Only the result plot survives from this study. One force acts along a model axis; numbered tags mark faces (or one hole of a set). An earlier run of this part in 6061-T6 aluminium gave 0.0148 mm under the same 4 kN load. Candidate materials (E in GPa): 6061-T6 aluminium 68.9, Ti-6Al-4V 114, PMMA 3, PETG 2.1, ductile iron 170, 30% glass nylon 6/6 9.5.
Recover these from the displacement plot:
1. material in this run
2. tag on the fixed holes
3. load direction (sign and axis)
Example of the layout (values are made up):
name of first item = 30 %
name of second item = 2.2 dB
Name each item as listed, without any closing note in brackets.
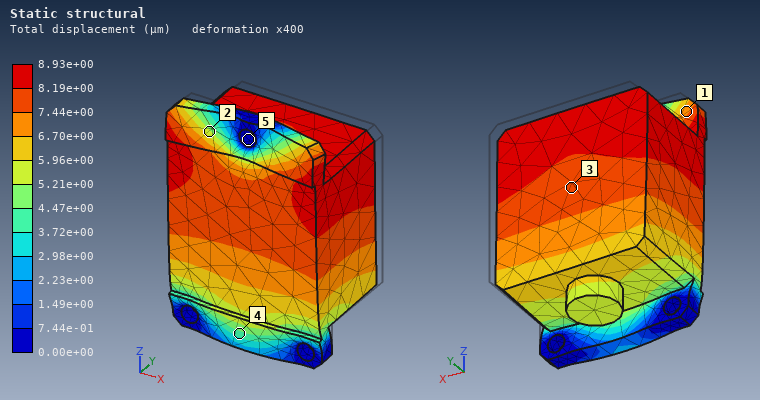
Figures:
material in this run = Ti-6Al-4V
tag on the fixed holes = 5
load direction = -Y
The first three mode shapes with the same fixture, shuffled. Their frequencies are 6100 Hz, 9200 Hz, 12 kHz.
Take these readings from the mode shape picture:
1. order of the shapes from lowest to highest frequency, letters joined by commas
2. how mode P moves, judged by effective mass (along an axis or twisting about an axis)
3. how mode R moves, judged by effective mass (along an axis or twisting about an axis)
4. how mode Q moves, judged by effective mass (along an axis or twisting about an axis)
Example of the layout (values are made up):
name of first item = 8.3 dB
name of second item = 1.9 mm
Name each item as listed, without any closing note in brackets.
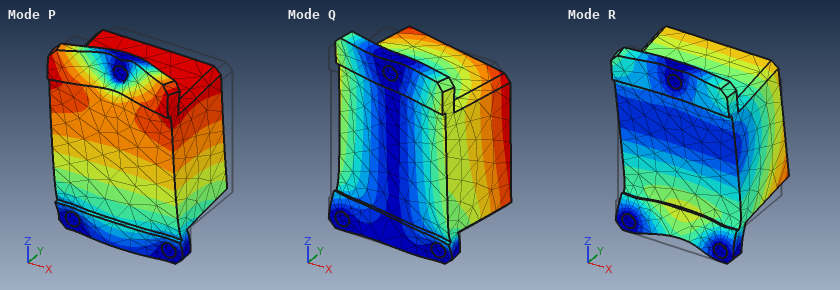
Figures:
order of the shapes from lowest to highest frequency, letters joined by commas = Q, P, R
how mode P moves, judged by effective mass = along Y
how mode R moves, judged by effective mass = along Z
how mode Q moves, judged by effective mass = along X
